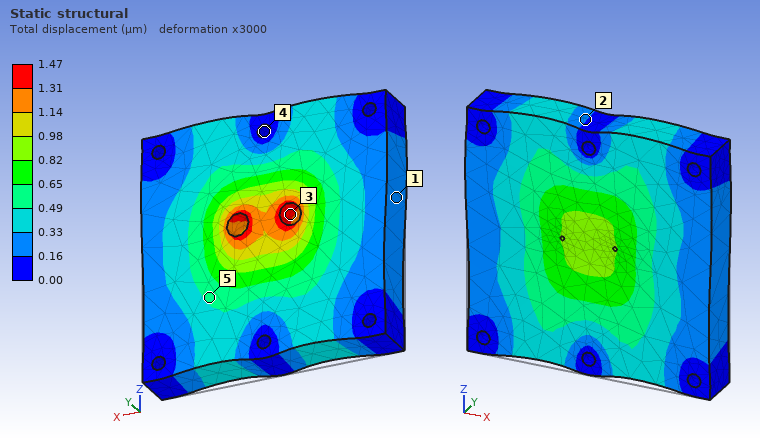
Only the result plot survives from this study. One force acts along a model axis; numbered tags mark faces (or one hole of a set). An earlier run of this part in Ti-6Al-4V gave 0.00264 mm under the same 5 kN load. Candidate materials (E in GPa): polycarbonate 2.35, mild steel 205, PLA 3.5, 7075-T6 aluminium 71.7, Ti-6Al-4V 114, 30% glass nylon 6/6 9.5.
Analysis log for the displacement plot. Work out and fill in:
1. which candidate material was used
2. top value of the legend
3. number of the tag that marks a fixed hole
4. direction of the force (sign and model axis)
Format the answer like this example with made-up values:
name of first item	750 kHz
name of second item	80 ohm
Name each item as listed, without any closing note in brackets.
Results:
which candidate material was used	mild steel
top value of the legend	1.47 µm
number of the tag that marks a fixed hole	4
direction of the force	+Z
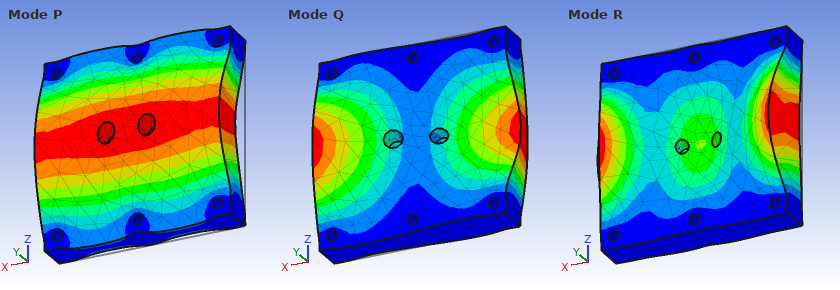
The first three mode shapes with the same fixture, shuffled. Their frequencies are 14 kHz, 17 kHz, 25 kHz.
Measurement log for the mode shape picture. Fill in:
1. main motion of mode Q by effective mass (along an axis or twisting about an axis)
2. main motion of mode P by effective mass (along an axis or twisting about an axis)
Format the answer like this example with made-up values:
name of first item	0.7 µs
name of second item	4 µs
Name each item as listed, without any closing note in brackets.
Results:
main motion of mode Q by effective mass	twisting about Z
main motion of mode P by effective mass	along Y
